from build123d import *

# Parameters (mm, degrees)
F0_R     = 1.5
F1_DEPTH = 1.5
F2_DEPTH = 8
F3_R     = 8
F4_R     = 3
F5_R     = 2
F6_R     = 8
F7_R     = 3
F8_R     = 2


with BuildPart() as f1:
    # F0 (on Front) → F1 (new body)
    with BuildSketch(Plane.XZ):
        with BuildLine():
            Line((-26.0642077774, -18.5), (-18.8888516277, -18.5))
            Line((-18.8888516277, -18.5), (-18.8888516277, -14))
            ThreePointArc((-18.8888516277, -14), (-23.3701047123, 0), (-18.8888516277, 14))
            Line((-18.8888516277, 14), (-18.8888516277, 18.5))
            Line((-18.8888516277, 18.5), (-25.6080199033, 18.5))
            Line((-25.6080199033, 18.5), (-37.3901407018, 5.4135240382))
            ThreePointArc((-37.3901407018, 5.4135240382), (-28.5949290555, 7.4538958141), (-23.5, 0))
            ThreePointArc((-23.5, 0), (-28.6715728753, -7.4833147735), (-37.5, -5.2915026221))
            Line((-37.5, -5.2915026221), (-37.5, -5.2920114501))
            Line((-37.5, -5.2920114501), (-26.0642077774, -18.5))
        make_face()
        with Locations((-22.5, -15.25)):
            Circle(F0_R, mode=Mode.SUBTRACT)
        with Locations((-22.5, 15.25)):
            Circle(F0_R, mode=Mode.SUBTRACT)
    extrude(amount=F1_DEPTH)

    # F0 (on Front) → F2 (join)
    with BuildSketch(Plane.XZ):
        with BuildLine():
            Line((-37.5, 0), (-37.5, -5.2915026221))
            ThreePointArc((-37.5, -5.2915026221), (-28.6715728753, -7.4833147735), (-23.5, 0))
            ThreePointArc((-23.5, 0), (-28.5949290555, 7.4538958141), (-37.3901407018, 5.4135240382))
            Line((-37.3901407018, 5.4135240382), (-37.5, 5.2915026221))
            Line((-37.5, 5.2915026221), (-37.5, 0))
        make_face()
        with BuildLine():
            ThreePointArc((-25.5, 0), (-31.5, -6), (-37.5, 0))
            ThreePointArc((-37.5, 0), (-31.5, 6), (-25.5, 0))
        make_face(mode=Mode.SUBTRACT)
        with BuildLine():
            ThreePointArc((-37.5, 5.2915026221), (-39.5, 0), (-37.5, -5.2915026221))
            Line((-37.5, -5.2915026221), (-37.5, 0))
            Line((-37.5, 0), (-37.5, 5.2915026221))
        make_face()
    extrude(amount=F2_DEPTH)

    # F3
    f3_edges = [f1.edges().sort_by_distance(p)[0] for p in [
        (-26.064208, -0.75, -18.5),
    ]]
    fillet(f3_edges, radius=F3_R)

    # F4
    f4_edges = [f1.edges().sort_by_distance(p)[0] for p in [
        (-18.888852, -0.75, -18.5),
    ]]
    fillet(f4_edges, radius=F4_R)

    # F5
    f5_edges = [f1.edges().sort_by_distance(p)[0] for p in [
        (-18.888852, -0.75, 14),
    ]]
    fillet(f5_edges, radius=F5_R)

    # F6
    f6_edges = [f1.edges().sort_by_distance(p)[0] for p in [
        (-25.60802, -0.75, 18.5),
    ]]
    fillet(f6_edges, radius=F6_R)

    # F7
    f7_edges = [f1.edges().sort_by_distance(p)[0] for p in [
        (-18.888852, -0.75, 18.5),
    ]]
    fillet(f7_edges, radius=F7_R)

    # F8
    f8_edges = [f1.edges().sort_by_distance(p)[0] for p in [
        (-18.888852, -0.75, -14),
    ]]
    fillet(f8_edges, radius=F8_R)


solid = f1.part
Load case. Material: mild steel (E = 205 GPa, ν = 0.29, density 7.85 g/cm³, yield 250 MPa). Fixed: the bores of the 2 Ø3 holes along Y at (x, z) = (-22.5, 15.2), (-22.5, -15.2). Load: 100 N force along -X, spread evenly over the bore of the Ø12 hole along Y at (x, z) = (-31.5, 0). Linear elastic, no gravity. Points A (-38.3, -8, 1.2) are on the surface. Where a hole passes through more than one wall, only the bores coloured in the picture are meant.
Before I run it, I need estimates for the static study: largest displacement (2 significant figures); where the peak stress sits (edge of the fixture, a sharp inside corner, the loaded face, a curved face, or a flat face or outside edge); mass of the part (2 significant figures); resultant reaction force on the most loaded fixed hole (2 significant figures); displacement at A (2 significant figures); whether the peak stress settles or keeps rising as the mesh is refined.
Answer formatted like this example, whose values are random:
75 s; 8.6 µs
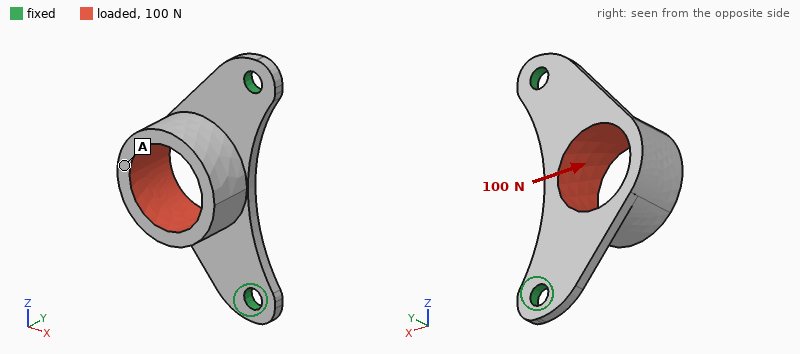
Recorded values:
31 µm; edge of the fixture; 8.4 g; 60 N; 29 µm; keeps rising
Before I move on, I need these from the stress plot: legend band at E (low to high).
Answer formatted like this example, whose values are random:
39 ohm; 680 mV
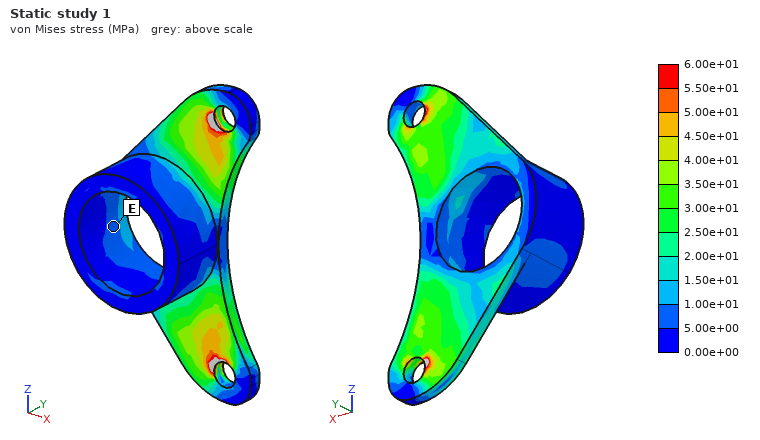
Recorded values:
5.00e+00 to 1.00e+01 MPa
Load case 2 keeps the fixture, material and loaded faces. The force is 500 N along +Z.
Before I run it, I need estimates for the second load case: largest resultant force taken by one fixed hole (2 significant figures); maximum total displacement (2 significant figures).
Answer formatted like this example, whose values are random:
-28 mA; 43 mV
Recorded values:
290 N; 14 µm
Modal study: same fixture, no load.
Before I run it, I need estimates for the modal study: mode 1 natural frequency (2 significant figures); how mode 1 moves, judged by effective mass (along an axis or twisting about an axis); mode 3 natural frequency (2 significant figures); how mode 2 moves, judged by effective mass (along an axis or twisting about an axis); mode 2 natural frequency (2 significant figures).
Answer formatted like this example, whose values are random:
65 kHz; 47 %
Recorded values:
3000 Hz; along Y; 11 kHz; along Y; 9500 Hz
